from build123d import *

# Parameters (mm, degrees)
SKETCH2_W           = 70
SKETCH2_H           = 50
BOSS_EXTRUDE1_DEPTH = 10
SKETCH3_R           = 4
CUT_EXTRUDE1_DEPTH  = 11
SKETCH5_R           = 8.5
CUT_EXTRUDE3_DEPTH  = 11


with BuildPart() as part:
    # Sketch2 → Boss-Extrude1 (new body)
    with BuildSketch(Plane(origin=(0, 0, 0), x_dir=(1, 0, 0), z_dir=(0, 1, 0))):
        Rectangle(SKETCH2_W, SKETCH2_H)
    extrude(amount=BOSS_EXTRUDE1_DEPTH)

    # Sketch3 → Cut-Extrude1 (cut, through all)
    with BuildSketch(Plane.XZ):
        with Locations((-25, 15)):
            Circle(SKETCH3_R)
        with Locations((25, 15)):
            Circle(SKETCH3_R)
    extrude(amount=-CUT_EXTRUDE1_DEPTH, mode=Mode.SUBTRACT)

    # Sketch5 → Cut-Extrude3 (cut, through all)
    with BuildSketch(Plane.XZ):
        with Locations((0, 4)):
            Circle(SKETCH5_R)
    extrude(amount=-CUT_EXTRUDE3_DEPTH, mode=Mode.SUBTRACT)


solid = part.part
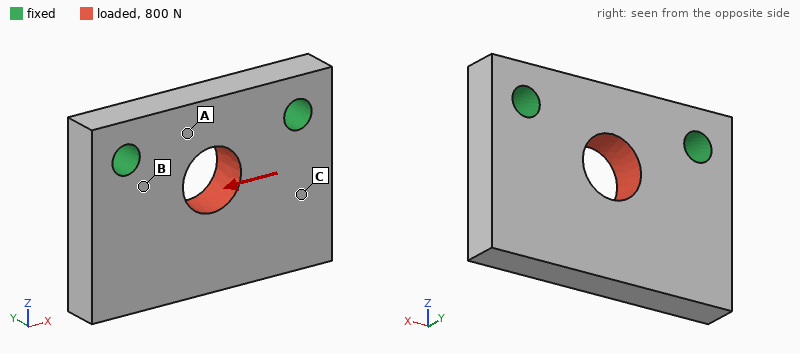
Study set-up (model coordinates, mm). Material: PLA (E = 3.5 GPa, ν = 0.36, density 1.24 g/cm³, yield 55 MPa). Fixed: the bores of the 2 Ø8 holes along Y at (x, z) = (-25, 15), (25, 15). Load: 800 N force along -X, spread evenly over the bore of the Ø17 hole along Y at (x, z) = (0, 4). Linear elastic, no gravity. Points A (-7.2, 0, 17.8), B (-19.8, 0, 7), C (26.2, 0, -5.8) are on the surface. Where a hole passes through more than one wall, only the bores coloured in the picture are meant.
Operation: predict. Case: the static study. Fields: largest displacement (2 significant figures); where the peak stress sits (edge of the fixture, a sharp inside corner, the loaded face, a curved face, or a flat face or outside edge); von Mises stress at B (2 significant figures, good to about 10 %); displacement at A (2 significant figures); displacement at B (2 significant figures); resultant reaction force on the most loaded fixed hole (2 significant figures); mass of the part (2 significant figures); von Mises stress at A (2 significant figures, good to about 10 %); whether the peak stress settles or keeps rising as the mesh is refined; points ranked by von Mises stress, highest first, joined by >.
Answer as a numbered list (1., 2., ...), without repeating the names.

1. 25 µm
2. edge of the fixture
3. 2.3 MPa
4. 5.0 µm
5. 7.9 µm
6. 420 N
7. 39 g
8. 1.2 MPa
9. keeps rising
10. B > A > C
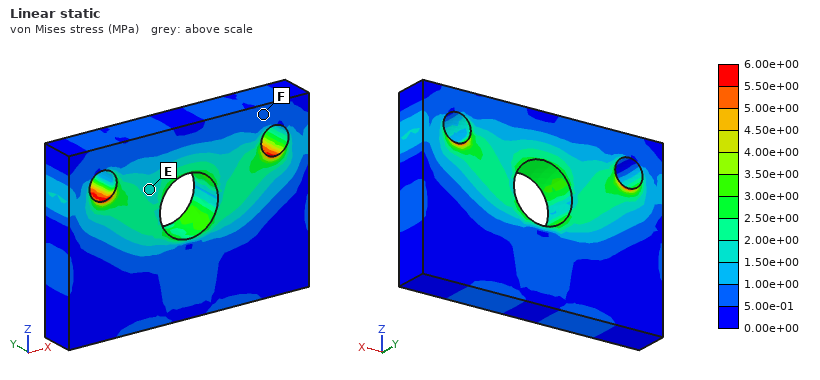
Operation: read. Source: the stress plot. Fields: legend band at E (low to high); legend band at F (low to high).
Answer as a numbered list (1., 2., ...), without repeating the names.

1. 1.50e+00 to 2.00e+00 MPa
2. 5.00e-01 to 1.00e+00 MPa
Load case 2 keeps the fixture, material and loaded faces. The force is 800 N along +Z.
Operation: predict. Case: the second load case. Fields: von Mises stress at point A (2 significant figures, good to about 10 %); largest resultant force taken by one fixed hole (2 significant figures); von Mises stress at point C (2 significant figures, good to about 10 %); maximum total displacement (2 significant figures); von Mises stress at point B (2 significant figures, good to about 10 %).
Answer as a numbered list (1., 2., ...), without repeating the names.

1. 1.7 MPa
2. 410 N
3. 0.86 MPa
4. 26 µm
5. 2.4 MPa
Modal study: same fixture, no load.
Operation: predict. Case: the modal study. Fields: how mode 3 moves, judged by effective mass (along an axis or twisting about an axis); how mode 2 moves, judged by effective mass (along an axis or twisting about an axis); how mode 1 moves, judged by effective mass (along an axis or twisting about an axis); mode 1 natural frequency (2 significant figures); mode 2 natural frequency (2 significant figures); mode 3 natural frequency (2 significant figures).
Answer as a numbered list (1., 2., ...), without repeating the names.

1. along X
2. twisting about Z
3. along Y
4. 1500 Hz
5. 2600 Hz
6. 4400 Hz
